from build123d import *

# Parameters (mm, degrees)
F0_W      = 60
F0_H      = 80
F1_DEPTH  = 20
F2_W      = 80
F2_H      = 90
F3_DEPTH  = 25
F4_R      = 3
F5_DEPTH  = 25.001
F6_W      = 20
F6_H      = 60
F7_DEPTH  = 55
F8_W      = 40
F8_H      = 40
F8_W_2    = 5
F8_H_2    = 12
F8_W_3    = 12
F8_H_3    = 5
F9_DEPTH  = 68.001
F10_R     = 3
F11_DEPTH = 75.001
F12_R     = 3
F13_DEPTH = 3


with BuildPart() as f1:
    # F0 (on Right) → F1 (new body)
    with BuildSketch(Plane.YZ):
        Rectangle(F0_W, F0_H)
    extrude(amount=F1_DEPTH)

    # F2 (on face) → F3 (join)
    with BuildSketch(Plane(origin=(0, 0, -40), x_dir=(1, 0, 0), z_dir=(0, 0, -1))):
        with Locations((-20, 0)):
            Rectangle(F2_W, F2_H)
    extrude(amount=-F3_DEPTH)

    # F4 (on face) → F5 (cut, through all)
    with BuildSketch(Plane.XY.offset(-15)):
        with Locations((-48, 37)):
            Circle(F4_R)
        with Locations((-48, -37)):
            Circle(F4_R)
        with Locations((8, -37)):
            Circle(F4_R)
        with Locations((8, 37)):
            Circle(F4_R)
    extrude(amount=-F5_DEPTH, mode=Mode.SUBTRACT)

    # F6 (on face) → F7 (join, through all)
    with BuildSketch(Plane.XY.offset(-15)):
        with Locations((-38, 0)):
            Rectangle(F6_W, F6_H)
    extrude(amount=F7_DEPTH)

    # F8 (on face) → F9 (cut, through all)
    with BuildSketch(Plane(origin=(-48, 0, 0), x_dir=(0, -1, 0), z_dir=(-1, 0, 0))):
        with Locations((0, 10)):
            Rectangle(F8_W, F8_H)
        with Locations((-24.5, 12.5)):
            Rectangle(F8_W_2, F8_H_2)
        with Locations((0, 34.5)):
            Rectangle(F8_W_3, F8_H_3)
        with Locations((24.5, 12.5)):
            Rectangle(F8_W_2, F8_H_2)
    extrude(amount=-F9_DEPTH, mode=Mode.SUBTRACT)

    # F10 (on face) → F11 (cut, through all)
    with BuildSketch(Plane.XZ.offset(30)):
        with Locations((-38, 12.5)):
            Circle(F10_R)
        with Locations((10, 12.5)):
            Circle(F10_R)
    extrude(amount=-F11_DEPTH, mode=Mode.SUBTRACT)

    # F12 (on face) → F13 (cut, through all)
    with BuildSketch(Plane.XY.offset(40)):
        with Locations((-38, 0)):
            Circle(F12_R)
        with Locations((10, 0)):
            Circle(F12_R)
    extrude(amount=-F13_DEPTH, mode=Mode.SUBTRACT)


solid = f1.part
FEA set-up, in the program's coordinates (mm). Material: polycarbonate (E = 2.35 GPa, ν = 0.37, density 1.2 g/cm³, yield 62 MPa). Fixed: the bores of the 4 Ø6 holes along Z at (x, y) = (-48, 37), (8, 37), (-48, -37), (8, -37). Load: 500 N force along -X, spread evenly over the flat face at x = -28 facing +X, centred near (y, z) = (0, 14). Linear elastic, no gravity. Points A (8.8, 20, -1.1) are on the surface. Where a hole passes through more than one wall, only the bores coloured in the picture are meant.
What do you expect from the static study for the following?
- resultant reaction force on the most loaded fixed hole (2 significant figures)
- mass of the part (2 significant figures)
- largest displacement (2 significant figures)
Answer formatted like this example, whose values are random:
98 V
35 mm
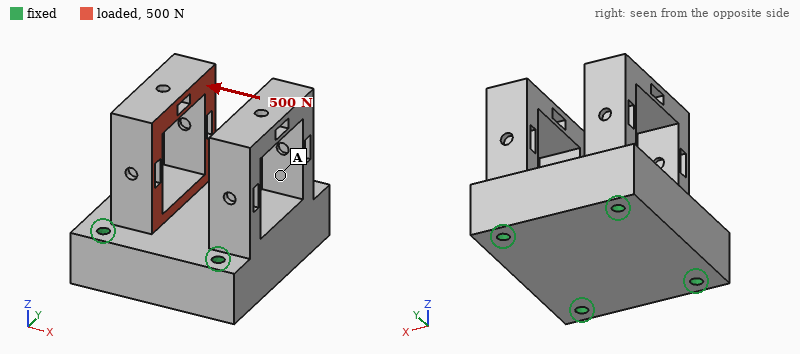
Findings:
220 N
280 g
0.69 mm
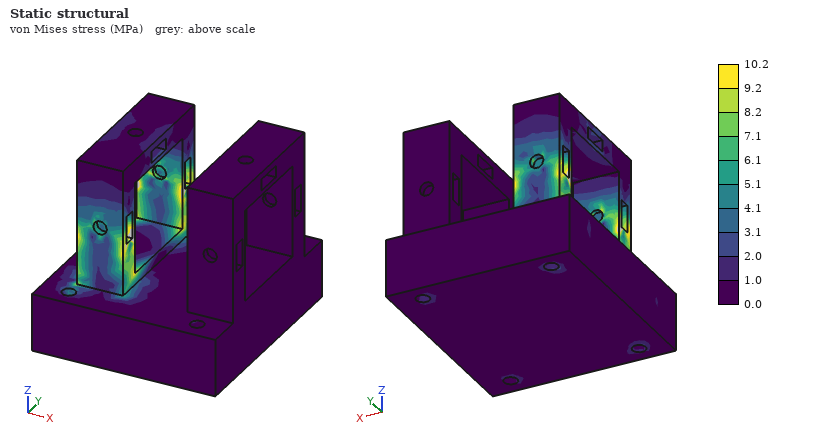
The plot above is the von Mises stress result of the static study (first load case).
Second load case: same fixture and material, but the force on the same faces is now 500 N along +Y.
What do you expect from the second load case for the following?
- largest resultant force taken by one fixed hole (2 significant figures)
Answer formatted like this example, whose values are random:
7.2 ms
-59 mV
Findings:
330 N
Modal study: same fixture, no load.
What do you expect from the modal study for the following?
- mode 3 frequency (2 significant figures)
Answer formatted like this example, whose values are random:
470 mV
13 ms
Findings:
790 Hz
